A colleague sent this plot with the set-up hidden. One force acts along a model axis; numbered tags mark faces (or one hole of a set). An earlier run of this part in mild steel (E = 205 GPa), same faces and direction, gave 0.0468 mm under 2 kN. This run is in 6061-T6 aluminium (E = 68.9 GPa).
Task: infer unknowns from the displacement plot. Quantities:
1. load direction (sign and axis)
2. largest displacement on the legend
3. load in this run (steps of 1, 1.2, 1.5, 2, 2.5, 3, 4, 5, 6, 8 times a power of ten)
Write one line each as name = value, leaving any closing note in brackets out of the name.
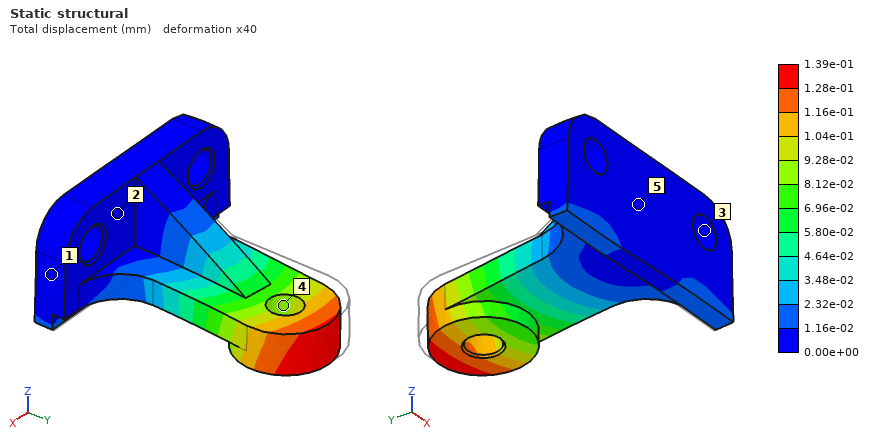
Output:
load direction = +X
largest displacement on the legend = 1.39e-01 mm
load in this run = 2 kN
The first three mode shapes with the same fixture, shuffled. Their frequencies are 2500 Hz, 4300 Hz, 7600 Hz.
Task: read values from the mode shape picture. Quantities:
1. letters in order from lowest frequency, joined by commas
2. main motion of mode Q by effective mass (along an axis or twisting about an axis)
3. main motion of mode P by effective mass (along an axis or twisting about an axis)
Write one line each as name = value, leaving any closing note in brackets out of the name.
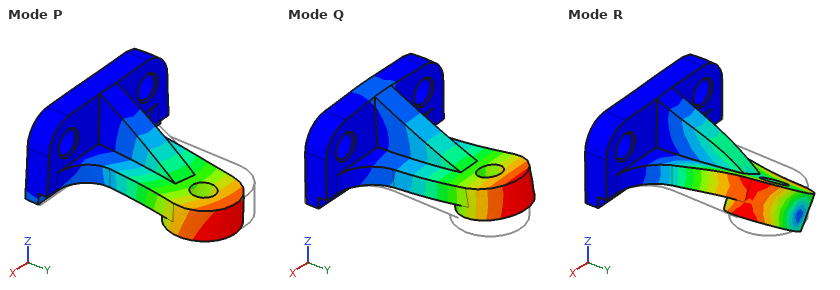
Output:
letters in order from lowest frequency, joined by commas = Q, P, R
main motion of mode Q by effective mass = along Z
main motion of mode P by effective mass = along X
